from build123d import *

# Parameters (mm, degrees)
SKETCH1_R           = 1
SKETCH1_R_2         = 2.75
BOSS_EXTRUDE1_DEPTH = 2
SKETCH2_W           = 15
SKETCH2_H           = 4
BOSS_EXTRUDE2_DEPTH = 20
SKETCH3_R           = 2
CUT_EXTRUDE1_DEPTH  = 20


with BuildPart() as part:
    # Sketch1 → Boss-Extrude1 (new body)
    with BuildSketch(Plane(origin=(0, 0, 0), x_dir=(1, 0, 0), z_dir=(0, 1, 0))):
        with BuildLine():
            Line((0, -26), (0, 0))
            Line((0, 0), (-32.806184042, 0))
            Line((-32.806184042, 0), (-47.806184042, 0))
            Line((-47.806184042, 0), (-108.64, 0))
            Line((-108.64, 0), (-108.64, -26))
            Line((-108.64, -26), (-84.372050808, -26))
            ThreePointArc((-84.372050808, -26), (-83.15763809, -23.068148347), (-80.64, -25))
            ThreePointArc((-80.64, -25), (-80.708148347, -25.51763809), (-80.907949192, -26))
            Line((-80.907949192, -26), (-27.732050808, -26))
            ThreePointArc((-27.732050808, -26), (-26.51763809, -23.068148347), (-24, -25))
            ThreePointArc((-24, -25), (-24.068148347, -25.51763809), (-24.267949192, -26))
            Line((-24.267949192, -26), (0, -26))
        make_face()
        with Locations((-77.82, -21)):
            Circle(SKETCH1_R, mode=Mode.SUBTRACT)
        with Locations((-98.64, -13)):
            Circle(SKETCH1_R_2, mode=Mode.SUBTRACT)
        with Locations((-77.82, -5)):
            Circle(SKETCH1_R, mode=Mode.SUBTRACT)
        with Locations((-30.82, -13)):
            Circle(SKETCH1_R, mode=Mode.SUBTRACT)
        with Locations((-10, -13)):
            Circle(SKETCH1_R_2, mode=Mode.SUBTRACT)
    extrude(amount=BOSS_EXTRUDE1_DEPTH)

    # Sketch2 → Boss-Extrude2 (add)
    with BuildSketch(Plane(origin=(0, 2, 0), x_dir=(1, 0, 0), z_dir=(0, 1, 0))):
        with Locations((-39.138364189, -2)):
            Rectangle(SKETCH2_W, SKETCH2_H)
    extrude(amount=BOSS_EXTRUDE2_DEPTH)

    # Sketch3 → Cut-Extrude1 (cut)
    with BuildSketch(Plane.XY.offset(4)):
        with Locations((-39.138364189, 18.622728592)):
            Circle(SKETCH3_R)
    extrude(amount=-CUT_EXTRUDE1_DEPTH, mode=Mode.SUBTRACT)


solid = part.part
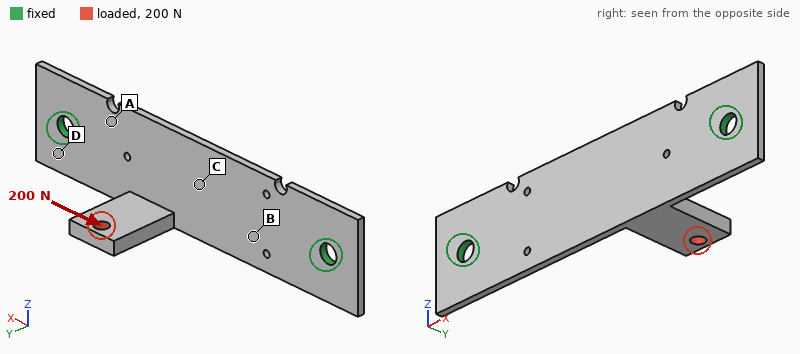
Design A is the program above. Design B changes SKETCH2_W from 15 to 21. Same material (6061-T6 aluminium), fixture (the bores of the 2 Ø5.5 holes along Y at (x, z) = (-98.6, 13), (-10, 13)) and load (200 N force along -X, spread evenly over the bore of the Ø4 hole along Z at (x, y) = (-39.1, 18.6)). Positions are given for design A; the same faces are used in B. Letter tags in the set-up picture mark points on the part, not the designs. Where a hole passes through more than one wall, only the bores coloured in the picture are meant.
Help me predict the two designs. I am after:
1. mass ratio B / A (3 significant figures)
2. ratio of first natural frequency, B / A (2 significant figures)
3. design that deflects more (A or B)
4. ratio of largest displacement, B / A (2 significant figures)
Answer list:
1.07
0.96
A
0.85
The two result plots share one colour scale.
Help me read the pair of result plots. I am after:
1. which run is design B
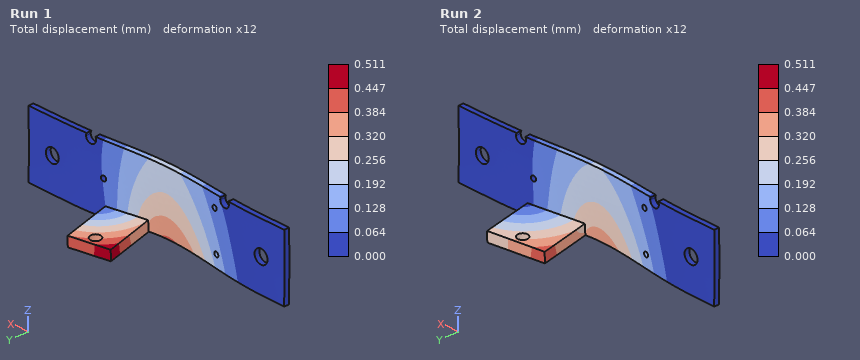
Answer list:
Run 2
